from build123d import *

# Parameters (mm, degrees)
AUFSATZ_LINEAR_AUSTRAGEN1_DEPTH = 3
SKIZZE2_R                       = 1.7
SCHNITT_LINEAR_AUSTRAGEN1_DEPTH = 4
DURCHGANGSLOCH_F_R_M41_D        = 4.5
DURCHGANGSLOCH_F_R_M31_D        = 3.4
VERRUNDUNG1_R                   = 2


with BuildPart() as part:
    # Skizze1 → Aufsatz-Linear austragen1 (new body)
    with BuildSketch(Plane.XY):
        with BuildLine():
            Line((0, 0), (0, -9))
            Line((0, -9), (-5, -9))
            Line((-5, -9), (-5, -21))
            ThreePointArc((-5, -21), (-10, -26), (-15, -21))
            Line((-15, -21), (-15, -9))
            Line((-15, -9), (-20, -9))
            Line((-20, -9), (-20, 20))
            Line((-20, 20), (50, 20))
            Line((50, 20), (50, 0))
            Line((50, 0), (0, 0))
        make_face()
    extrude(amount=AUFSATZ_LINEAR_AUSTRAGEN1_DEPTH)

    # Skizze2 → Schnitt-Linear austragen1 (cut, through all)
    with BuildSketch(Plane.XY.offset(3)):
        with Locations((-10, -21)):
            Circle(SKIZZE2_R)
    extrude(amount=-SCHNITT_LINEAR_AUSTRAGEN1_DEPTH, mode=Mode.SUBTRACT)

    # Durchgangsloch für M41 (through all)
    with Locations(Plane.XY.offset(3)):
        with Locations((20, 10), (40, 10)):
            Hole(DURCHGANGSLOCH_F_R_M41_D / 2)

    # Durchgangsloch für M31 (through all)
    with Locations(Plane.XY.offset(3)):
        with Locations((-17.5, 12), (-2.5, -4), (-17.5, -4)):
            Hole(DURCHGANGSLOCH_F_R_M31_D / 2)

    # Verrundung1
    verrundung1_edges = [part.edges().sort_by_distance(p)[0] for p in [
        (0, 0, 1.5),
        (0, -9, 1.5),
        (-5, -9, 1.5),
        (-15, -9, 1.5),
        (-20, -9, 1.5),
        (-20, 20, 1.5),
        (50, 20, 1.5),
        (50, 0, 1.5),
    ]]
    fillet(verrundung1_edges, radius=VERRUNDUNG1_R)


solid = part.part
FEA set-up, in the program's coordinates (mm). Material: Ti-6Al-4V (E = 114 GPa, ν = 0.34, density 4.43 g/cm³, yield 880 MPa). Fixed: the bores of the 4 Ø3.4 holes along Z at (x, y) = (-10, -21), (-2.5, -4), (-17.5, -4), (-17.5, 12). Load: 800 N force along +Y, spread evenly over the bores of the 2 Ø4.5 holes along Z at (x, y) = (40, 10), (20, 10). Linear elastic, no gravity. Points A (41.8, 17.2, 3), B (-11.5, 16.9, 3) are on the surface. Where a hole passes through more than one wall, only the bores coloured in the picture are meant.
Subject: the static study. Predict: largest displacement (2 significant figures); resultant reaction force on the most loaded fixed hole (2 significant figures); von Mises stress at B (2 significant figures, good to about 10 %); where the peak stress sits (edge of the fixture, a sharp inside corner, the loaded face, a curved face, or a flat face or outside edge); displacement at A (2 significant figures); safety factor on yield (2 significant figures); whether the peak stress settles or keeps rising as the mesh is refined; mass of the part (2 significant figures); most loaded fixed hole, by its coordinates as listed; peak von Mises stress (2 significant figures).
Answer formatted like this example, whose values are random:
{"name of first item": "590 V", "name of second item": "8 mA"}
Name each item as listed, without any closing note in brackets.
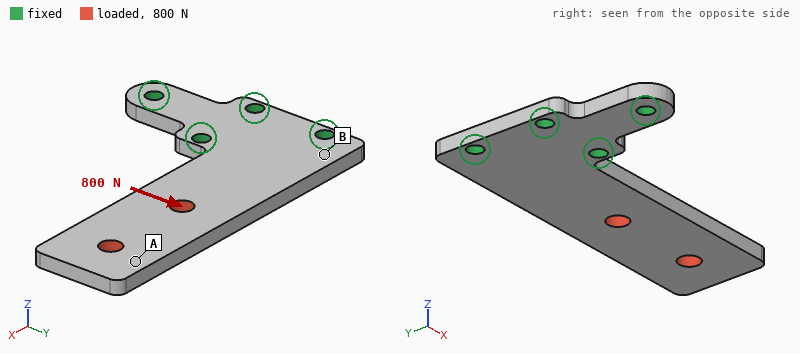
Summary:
{"largest displacement": "0.13 mm", "resultant reaction force on the most loaded fixed hole": "1.5 kN", "von Mises stress at B": "56 MPa", "where the peak stress sits": "a curved face", "displacement at A": "0.11 mm", "safety factor on yield": "2.4", "whether the peak stress settles or keeps rising as the mesh is refined": "settles", "mass of the part": "22 g", "most loaded fixed hole, by its coordinates as listed": "(-2.5, -4)", "peak von Mises stress": "360 MPa"}
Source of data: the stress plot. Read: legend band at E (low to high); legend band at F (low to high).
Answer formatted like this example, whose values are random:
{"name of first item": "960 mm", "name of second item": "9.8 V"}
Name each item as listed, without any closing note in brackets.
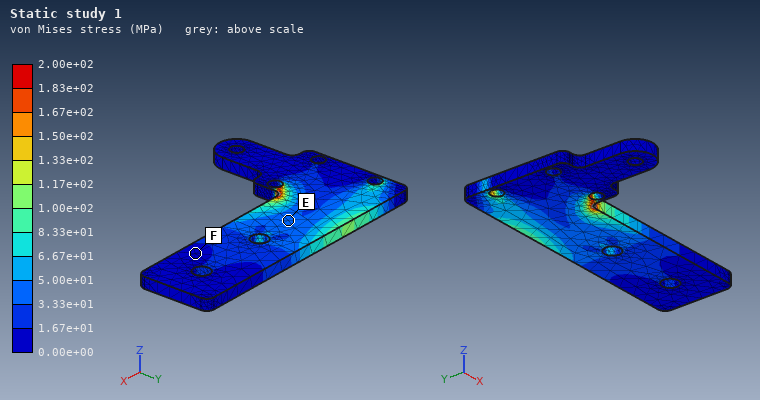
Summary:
{"legend band at E": "3.33e+01 to 5.00e+01 MPa", "legend band at F": "0.00e+00 to 1.67e+01 MPa"}
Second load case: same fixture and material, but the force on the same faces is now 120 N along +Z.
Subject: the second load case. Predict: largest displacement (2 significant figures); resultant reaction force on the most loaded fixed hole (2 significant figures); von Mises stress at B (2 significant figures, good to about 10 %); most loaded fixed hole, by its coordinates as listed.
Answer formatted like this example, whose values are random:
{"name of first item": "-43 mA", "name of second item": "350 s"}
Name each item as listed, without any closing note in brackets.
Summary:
{"largest displacement": "0.83 mm", "resultant reaction force on the most loaded fixed hole": "270 N", "von Mises stress at B": "59 MPa", "most loaded fixed hole, by its coordinates as listed": "(-2.5, -4)"}
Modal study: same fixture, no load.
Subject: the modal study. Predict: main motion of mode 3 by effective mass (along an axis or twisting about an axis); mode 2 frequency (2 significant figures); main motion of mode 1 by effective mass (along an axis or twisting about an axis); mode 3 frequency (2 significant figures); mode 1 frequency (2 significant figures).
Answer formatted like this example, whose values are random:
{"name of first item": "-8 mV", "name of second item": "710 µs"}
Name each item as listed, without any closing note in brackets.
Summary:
{"main motion of mode 3 by effective mass": "along Y", "mode 2 frequency": "3500 Hz", "main motion of mode 1 by effective mass": "along Z", "mode 3 frequency": "4600 Hz", "mode 1 frequency": "740 Hz"}
